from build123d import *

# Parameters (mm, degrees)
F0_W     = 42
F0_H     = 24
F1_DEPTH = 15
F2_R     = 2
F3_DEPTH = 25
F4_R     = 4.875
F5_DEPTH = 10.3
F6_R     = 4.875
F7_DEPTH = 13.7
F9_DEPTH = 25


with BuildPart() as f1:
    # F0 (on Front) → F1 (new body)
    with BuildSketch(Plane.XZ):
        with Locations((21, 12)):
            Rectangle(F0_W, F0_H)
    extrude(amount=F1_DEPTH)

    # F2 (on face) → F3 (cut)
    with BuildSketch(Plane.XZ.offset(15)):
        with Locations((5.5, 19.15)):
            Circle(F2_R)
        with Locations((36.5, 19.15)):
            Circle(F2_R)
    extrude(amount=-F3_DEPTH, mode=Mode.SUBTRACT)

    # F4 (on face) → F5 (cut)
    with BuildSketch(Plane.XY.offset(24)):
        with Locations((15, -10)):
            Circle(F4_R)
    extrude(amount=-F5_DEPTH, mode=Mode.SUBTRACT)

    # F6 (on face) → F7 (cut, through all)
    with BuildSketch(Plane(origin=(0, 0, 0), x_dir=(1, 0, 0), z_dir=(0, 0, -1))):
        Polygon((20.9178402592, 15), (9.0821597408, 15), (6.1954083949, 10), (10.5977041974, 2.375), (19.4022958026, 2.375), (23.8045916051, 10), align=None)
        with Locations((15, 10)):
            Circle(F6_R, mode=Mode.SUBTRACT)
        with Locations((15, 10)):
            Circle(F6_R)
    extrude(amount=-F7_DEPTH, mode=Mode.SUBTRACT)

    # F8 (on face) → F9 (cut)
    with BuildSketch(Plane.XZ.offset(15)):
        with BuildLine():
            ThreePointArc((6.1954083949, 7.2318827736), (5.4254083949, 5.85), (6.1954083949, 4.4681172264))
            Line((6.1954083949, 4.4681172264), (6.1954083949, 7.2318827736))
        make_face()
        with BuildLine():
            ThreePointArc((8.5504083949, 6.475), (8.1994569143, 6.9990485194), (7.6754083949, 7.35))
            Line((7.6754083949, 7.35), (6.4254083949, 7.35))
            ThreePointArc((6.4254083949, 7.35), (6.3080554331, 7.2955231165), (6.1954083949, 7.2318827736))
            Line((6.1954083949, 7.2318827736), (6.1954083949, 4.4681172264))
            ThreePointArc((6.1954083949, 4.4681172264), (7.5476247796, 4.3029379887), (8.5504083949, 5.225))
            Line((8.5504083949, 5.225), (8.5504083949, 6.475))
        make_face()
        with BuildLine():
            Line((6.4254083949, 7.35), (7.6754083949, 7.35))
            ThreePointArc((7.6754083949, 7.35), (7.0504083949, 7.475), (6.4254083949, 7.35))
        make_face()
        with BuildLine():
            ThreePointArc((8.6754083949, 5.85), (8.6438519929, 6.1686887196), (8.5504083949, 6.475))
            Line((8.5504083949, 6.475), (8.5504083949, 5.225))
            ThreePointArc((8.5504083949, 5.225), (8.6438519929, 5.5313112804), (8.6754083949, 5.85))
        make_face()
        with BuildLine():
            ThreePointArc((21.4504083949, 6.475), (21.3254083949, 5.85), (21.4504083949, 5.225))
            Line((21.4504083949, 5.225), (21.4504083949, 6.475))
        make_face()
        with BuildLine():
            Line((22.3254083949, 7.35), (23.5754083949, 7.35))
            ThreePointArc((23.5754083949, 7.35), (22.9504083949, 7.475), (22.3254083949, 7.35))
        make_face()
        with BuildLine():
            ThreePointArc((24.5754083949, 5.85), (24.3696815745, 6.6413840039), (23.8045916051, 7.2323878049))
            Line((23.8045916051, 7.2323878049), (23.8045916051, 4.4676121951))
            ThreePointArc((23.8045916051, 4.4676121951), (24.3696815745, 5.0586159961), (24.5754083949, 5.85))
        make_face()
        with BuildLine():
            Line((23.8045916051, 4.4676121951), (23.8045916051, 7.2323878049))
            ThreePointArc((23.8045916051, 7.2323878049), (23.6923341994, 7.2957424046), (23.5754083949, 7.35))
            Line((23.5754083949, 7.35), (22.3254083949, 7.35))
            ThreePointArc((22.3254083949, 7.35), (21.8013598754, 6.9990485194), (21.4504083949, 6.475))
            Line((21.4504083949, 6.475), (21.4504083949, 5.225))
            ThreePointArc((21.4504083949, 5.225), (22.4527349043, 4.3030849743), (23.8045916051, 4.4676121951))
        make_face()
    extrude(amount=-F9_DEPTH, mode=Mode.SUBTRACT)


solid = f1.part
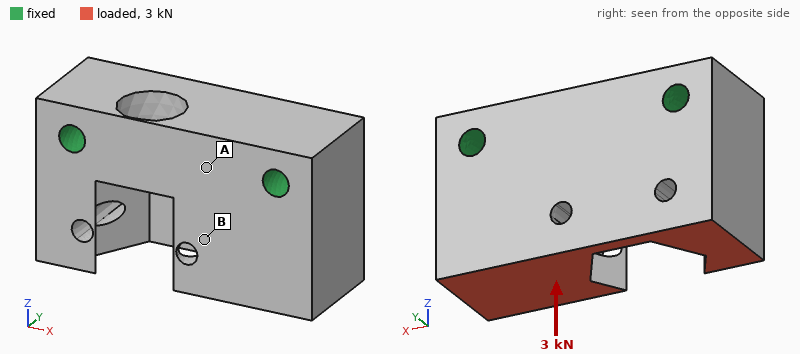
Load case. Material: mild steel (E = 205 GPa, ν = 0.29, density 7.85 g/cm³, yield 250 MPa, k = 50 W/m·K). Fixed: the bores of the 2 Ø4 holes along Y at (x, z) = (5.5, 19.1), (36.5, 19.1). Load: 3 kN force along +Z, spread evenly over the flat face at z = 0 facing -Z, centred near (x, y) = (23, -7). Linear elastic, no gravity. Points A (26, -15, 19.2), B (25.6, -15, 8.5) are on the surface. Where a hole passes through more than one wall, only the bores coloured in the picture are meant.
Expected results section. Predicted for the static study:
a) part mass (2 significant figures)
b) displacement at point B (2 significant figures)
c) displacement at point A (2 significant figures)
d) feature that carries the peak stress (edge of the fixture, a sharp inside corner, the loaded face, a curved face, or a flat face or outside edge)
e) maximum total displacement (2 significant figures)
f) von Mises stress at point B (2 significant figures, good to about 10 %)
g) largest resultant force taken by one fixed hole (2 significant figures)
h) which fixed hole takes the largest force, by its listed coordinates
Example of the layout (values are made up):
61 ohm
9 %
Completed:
89 g
1.1 µm
0.79 µm
a curved face
2.1 µm
8.3 MPa
1.8 kN
(36.5, 19.1)
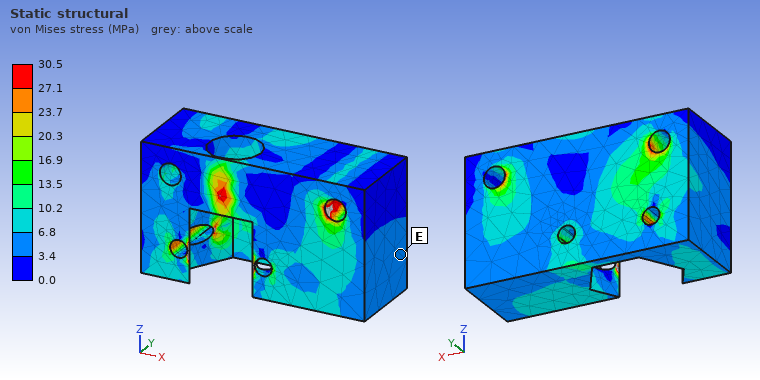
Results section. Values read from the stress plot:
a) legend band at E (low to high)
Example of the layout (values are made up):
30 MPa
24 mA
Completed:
3.4 to 6.8 MPa
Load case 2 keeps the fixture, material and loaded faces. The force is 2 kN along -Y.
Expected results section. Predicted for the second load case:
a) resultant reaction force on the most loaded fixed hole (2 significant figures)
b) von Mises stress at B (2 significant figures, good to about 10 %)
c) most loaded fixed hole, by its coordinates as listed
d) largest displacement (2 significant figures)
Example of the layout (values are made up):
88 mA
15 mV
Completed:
1.3 kN
16 MPa
(36.5, 19.1)
7.7 µm
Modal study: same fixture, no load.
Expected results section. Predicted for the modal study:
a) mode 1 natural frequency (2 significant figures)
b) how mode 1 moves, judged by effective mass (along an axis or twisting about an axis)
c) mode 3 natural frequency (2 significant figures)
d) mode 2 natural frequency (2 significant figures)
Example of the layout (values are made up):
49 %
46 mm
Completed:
19 kHz
along Y
25 kHz
22 kHz
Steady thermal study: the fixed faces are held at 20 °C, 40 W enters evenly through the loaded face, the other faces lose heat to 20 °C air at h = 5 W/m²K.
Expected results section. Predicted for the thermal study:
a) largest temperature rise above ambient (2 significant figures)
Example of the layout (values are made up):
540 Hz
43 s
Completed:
40 K
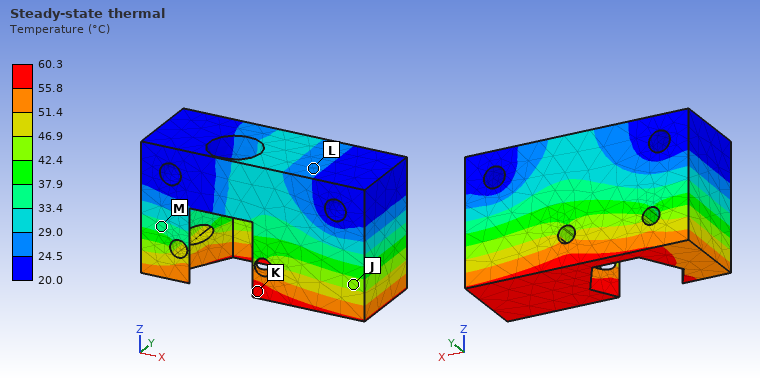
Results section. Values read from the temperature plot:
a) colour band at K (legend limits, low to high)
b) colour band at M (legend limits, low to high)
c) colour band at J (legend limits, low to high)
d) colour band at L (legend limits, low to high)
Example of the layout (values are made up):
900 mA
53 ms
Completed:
55.8 to 60.3 °C
33.4 to 37.9 °C
42.4 to 46.9 °C
24.5 to 29.0 °C
